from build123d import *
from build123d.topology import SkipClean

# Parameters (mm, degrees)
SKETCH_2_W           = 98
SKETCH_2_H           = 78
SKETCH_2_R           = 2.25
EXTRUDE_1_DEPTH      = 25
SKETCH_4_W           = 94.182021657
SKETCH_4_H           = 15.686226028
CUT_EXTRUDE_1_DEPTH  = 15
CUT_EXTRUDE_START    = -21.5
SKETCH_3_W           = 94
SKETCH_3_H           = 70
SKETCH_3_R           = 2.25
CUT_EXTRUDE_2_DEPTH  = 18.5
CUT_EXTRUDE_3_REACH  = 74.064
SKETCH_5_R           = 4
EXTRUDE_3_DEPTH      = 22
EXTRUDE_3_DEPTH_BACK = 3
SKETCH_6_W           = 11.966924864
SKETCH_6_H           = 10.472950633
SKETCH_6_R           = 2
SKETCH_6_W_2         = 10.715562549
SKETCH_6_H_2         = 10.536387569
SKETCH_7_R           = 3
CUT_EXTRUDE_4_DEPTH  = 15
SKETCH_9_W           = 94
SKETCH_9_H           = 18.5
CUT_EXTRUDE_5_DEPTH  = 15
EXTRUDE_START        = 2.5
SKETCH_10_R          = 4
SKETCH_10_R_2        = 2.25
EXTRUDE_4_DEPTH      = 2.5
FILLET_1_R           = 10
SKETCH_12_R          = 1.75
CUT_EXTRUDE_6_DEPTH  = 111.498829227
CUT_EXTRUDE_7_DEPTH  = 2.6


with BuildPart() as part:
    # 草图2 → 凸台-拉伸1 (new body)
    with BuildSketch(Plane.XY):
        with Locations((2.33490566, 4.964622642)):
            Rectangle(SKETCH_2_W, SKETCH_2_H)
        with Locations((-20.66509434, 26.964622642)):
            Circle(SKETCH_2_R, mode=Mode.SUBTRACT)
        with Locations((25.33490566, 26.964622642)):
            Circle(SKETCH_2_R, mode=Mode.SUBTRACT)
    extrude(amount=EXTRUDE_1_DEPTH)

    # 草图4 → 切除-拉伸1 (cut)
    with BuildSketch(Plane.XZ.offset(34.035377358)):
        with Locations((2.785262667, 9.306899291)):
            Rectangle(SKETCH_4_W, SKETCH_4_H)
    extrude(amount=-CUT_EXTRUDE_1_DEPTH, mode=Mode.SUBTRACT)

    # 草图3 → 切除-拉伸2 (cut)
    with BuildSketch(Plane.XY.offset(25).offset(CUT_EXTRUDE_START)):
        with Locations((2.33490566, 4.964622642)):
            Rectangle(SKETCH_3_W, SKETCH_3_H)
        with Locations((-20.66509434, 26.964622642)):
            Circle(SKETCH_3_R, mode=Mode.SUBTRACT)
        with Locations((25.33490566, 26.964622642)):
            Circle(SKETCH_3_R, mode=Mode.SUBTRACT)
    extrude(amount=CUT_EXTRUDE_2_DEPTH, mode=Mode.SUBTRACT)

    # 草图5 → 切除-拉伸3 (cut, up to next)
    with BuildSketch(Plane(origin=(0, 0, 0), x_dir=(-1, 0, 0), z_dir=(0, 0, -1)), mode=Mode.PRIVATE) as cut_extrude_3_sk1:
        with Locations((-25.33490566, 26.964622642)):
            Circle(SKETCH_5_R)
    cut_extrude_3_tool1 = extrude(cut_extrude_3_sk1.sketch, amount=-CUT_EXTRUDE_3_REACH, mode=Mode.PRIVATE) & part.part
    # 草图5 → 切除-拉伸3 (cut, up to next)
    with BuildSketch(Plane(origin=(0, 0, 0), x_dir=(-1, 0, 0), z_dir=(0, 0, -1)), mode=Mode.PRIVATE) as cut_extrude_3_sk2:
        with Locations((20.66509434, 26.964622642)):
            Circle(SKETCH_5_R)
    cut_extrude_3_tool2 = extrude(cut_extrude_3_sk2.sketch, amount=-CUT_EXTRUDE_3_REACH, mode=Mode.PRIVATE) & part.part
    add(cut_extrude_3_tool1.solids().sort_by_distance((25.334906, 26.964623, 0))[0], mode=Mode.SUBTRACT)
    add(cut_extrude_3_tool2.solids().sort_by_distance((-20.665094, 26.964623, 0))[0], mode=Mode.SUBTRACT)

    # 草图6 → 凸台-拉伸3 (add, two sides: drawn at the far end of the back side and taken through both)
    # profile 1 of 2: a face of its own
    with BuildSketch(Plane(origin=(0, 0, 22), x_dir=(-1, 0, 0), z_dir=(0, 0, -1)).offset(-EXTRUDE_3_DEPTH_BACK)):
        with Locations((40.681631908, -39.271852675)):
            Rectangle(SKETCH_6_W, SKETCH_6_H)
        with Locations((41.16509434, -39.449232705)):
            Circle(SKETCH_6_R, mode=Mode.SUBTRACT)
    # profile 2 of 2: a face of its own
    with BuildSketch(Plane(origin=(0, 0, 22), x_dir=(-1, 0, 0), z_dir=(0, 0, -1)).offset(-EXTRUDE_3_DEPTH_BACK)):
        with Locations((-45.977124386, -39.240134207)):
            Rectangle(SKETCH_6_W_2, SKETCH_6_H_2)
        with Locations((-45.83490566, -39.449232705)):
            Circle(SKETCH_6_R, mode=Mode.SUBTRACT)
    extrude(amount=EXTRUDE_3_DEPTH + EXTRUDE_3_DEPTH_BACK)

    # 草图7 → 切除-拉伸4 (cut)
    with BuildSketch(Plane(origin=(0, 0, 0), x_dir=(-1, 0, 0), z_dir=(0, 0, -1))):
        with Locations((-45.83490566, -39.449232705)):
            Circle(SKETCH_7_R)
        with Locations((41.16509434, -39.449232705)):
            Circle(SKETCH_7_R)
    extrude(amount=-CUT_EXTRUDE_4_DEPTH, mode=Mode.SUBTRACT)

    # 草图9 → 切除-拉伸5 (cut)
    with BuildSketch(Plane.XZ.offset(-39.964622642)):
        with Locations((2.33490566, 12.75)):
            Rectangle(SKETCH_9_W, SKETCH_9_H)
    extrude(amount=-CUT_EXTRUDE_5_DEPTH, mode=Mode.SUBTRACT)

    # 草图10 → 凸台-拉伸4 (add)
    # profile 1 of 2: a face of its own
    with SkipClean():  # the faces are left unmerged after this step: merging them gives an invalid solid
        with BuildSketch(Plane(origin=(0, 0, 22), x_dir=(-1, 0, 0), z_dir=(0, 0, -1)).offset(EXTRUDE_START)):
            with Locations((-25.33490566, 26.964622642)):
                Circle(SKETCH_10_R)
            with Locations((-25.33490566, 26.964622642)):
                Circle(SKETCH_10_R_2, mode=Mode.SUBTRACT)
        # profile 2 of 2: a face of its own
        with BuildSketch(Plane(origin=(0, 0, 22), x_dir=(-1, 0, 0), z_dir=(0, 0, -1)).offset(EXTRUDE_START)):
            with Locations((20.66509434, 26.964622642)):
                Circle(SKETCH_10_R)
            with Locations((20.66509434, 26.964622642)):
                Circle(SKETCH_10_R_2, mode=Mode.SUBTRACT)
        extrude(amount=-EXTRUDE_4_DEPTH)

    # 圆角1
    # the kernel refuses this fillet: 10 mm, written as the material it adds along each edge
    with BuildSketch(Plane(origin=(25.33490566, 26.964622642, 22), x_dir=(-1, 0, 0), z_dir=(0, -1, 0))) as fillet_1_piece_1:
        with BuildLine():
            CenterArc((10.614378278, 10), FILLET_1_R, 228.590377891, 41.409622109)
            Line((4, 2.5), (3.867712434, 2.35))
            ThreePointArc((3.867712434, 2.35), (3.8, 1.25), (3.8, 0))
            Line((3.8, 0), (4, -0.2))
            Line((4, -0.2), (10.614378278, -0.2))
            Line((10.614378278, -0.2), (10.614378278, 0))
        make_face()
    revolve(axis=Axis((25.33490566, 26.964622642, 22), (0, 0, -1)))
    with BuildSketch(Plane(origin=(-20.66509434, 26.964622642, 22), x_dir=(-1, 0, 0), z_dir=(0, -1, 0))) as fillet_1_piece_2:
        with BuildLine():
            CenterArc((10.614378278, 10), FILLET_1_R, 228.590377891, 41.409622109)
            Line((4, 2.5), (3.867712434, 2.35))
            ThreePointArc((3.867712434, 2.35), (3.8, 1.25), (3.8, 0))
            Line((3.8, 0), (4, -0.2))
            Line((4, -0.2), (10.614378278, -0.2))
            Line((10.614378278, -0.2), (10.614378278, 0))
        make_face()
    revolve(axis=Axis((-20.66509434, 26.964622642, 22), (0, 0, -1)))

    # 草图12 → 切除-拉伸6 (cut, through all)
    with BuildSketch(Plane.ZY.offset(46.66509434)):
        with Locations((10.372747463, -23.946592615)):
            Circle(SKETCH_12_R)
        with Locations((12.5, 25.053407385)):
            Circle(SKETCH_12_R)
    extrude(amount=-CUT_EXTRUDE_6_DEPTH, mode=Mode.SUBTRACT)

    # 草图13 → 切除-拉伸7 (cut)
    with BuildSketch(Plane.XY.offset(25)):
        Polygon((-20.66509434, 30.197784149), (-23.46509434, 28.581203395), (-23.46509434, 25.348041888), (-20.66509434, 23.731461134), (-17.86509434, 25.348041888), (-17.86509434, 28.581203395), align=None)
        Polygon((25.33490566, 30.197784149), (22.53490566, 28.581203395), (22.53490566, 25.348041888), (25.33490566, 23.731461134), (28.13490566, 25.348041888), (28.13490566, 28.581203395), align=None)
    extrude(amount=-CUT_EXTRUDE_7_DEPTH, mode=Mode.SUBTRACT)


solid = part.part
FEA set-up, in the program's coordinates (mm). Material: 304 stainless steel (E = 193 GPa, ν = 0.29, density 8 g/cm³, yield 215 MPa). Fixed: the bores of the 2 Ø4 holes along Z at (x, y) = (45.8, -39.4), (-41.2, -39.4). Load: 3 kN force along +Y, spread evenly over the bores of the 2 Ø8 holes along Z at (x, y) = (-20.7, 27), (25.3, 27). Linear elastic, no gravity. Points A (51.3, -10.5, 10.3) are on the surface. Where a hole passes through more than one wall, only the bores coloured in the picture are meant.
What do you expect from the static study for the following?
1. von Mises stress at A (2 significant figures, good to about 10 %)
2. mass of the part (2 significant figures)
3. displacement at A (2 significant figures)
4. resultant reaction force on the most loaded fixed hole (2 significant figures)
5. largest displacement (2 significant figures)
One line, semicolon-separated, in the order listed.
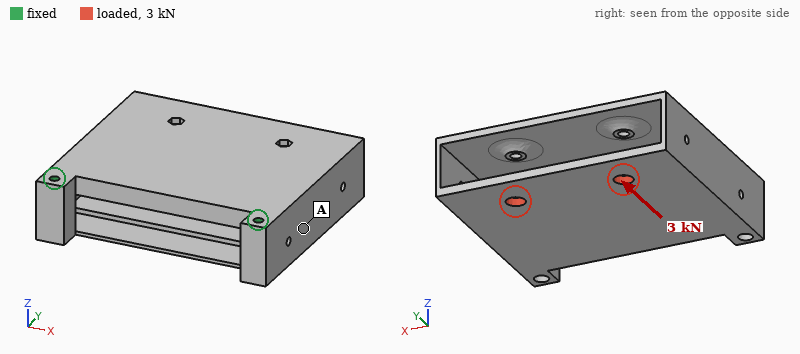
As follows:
14 MPa; 470 g; 27 µm; 1.5 kN; 89 µm
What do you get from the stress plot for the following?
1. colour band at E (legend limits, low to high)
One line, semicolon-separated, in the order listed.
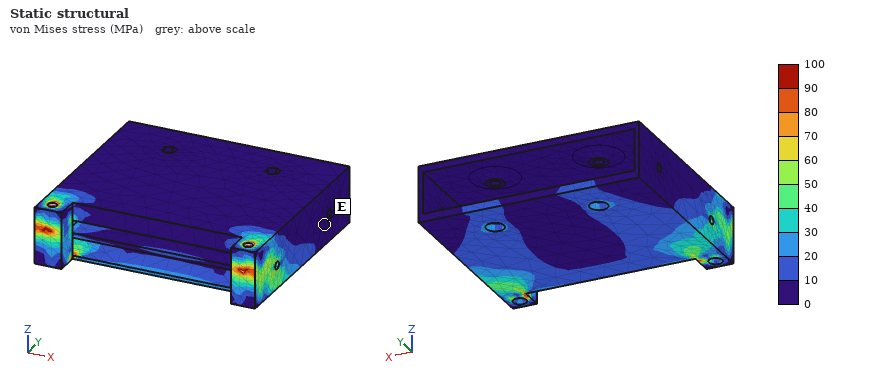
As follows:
0 to 10 MPa
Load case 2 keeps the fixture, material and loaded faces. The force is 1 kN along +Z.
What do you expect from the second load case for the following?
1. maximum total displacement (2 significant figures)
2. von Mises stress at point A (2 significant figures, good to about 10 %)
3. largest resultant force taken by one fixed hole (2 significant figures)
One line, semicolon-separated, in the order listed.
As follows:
0.32 mm; 41 MPa; 530 N
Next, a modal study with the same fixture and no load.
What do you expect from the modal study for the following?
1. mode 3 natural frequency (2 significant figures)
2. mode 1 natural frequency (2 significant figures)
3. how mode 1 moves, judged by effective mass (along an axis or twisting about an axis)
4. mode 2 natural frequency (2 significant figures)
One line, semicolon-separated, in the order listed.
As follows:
1700 Hz; 920 Hz; along Z; 1200 Hz
